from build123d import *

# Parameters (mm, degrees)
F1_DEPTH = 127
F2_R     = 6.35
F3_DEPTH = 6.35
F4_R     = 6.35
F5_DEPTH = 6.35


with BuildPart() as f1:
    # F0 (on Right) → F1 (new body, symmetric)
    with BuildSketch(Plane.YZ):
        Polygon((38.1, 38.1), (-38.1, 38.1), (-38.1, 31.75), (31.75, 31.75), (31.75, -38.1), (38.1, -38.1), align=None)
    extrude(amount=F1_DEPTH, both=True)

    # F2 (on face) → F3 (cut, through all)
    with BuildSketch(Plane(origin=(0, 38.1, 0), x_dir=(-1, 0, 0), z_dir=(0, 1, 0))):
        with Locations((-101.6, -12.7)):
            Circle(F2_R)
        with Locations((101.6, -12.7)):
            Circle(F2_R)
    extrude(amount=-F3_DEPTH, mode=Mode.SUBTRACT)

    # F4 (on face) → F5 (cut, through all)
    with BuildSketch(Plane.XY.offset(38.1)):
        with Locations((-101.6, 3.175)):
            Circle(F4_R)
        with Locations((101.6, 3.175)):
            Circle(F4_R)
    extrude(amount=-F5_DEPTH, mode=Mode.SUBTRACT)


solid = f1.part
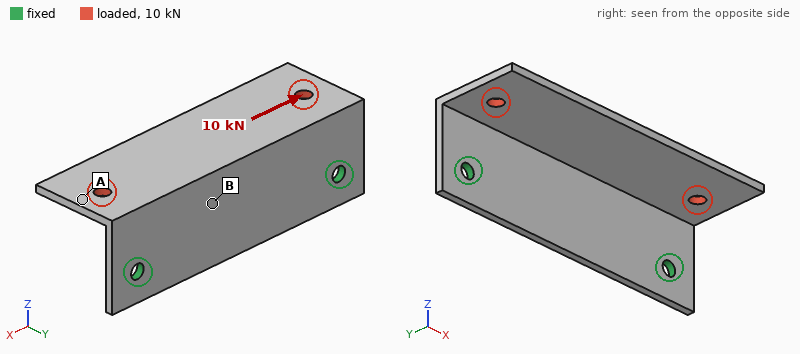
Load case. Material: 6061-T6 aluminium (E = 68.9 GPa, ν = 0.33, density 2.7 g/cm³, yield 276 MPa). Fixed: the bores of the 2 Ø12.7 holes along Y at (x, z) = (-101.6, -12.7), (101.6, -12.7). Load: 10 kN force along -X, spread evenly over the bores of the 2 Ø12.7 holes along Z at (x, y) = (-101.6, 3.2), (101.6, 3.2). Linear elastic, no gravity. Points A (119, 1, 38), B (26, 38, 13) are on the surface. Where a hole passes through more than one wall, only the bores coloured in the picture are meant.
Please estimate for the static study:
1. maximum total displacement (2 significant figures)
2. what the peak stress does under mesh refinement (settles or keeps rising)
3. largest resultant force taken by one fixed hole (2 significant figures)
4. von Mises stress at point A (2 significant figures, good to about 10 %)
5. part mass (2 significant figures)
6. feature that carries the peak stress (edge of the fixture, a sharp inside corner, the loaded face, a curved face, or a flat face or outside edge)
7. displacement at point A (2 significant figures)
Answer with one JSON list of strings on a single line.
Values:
["0.75 mm", "keeps rising", "5.7 kN", "29 MPa", "630 g", "edge of the fixture", "0.53 mm"]
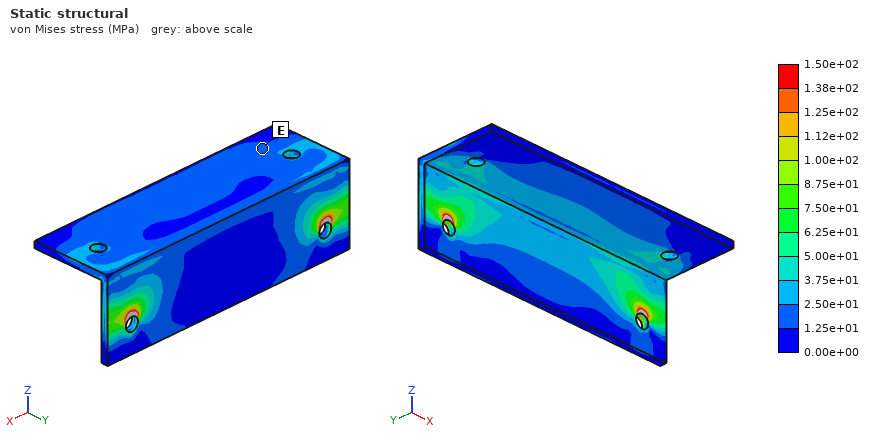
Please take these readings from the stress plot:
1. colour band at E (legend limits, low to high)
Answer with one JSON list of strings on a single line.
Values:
["1.25e+01 to 2.50e+01 MPa"]
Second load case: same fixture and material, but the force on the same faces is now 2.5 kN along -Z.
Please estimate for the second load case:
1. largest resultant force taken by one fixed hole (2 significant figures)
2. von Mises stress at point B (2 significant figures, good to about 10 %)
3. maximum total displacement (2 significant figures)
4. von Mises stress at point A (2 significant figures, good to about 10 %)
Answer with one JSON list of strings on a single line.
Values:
["1.3 kN", "21 MPa", "1.3 mm", "20 MPa"]
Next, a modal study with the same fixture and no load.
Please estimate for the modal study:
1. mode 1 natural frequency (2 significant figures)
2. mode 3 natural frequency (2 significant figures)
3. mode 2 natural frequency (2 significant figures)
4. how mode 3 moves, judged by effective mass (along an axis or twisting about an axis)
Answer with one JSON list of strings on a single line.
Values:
["410 Hz", "960 Hz", "700 Hz", "along Y"]
